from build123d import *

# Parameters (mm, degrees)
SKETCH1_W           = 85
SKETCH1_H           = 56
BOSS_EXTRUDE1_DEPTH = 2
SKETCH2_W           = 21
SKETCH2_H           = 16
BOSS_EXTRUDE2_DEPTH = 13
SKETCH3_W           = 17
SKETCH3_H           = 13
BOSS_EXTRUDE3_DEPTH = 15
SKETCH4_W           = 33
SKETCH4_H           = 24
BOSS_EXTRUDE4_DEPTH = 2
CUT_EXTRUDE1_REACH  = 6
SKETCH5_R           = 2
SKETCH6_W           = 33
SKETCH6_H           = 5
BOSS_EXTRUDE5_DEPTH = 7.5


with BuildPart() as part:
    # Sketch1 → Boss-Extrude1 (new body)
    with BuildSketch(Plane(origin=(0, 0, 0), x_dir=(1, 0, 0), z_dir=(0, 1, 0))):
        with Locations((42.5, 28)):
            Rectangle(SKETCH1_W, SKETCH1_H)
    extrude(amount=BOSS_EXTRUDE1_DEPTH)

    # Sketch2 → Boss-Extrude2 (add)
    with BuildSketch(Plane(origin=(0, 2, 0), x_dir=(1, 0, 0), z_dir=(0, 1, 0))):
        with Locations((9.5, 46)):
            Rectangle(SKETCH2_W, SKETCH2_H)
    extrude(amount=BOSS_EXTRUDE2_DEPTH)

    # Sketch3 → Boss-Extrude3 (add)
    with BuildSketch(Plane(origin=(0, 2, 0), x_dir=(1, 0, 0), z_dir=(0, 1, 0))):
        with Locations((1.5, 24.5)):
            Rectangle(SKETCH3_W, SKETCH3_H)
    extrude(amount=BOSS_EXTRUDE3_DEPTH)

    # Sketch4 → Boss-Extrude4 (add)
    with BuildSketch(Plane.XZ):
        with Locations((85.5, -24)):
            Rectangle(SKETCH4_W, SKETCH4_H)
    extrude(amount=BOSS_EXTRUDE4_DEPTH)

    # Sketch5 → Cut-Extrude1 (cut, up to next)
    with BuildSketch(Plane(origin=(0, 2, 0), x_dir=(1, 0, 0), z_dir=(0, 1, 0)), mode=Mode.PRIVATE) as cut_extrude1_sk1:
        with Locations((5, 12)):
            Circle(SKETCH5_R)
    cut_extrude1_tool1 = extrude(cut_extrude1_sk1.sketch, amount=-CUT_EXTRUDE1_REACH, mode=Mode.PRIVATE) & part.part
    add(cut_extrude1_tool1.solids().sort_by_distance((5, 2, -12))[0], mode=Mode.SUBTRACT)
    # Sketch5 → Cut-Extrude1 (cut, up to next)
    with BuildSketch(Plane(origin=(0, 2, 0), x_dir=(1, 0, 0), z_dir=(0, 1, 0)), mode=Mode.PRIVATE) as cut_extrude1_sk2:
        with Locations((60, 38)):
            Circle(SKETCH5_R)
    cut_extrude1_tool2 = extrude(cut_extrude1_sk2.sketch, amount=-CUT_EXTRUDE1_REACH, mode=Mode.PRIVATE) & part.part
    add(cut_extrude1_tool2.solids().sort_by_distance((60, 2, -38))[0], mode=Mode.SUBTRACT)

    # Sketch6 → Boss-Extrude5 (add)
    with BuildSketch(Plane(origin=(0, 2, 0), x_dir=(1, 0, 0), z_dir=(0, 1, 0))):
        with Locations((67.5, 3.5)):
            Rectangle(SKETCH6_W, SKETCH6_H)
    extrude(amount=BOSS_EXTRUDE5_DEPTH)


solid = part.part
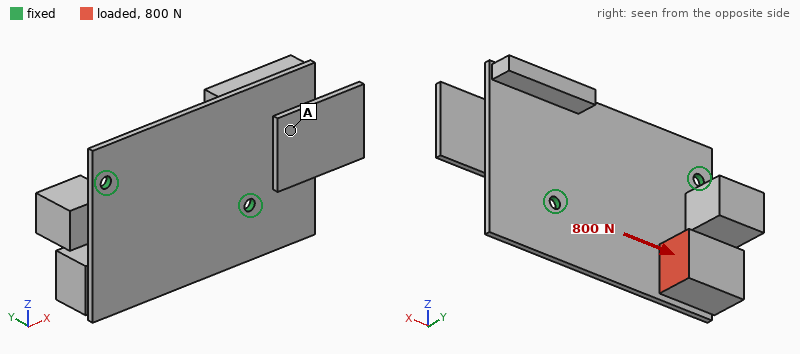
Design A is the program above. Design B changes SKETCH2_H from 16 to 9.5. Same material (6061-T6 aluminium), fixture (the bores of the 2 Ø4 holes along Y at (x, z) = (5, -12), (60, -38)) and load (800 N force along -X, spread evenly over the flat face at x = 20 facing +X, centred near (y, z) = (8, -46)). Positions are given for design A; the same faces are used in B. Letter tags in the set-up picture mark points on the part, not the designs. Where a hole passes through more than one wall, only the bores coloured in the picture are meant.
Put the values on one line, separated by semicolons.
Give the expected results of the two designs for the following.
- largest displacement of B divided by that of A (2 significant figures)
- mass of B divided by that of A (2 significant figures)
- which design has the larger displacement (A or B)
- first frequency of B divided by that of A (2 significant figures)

1.2; 0.91; B; 1.1
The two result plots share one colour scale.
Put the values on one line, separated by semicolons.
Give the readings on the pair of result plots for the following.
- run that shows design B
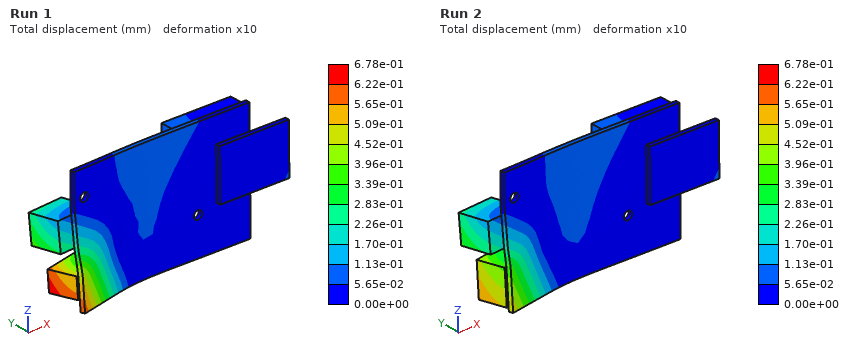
Run 1
